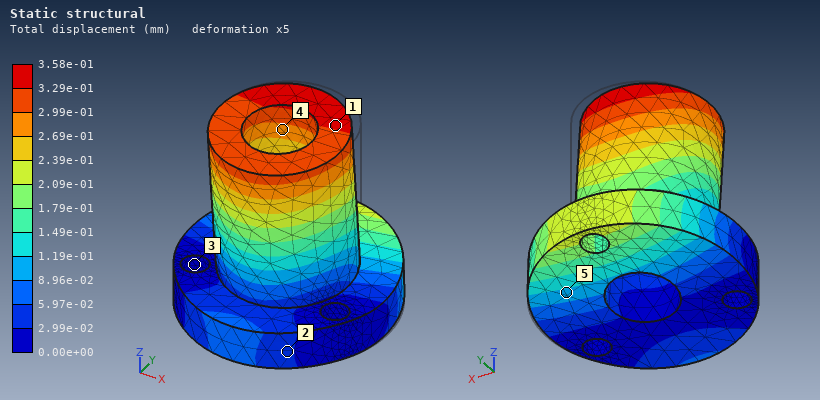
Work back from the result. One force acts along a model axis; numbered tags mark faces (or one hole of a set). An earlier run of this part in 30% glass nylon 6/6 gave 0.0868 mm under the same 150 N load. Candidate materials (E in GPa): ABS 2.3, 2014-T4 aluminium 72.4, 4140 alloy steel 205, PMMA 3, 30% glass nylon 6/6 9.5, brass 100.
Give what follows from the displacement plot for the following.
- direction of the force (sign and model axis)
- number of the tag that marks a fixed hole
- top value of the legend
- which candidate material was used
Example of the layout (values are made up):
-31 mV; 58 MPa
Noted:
-Y; 3; 3.58e-01 mm; ABS
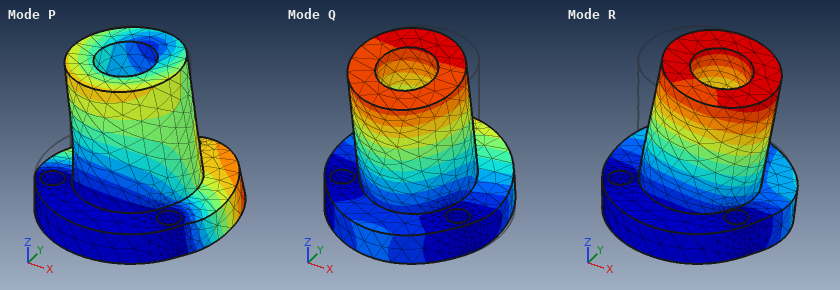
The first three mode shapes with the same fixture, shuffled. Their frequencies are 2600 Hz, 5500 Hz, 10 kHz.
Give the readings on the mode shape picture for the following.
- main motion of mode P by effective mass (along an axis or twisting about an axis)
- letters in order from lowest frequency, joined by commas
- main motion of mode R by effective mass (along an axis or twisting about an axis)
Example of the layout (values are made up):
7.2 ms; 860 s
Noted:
along X; Q, R, P; along X
